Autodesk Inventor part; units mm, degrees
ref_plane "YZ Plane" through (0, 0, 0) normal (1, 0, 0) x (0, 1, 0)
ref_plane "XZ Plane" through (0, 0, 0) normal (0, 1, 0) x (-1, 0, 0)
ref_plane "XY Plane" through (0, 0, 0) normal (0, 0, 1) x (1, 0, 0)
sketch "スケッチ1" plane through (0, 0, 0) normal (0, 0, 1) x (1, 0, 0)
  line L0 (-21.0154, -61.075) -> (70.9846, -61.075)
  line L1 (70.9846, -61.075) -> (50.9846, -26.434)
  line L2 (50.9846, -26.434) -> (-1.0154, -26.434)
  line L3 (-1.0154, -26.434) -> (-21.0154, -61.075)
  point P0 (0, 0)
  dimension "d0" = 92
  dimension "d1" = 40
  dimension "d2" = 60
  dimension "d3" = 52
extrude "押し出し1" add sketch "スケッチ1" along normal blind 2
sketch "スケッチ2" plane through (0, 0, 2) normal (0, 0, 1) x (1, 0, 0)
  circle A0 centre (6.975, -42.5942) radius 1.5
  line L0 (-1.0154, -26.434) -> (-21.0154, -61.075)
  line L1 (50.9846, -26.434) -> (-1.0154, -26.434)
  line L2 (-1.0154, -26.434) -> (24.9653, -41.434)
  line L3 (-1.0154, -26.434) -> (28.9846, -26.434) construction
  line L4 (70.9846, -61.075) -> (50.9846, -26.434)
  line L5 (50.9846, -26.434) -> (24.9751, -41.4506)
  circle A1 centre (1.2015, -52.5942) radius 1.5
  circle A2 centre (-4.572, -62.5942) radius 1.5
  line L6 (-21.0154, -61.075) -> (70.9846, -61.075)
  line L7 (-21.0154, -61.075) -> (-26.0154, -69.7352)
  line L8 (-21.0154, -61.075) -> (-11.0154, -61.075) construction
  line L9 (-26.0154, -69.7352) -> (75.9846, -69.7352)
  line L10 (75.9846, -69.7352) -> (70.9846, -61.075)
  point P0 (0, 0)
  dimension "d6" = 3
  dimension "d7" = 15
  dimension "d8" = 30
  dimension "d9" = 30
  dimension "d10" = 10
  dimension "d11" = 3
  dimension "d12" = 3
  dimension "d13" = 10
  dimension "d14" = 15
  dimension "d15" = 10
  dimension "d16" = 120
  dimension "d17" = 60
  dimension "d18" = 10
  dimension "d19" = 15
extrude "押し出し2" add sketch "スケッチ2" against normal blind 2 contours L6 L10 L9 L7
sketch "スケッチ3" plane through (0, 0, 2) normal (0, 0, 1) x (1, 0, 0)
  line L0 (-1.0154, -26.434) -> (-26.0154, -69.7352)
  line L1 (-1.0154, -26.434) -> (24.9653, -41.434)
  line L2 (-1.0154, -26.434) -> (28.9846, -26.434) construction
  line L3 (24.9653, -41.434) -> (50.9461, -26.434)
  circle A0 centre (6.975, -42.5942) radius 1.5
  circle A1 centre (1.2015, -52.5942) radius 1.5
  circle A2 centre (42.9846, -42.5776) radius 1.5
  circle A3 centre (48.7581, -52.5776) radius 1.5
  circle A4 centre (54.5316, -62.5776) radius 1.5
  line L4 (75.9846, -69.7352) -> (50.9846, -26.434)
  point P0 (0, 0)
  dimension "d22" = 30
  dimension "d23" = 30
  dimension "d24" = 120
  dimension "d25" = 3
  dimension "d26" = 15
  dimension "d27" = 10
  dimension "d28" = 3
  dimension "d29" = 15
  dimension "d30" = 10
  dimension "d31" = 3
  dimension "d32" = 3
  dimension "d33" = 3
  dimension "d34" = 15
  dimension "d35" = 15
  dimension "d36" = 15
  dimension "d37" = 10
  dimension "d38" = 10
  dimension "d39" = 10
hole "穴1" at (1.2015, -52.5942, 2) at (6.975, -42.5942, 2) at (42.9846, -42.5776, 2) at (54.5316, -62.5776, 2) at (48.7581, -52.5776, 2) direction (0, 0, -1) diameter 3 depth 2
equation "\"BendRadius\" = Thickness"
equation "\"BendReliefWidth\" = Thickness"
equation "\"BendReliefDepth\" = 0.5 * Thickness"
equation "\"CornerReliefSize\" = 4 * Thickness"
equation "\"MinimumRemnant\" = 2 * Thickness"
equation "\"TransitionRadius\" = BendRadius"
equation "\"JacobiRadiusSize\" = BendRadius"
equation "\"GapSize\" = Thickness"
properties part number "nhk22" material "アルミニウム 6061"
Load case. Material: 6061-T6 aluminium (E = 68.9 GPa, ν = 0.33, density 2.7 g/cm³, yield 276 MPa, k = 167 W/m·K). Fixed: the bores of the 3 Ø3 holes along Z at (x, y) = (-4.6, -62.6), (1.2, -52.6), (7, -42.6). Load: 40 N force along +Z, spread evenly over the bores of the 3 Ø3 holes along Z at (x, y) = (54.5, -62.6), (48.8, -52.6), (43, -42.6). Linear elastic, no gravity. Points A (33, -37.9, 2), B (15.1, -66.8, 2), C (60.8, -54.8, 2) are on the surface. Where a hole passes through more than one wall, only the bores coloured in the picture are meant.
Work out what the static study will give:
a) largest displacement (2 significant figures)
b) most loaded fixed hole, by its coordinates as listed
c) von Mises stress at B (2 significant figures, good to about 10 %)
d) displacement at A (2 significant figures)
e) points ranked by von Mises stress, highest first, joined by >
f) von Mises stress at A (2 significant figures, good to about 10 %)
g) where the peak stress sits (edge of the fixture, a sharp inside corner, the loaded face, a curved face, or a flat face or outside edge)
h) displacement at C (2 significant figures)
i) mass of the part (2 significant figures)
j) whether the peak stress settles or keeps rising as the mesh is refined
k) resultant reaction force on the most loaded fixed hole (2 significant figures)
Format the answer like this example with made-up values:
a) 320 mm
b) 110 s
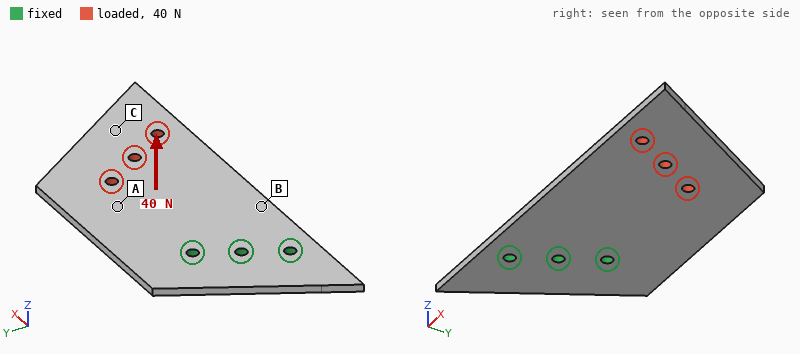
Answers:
a) 1.2 mm
b) (7, -42.6)
c) 40 MPa
d) 0.25 mm
e) B > A > C
f) 22 MPa
g) edge of the fixture
h) 0.83 mm
i) 18 g
j) keeps rising
k) 50 N
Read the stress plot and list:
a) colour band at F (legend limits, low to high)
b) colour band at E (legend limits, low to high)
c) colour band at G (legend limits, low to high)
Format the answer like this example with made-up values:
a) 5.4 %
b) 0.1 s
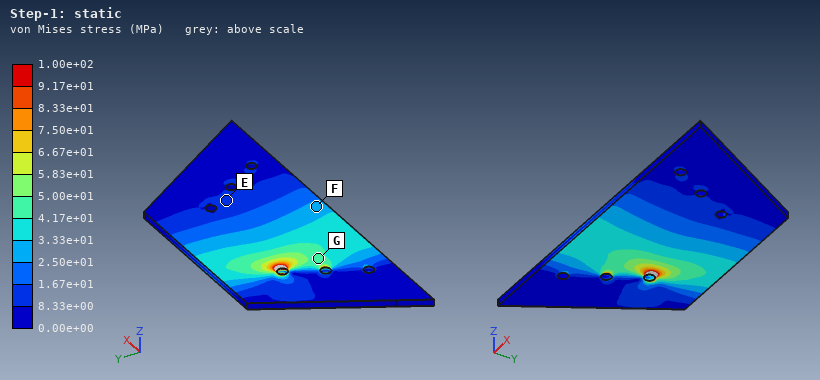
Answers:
a) 2.50e+01 to 3.33e+01 MPa
b) 8.33e+00 to 1.67e+01 MPa
c) 4.17e+01 to 5.00e+01 MPa
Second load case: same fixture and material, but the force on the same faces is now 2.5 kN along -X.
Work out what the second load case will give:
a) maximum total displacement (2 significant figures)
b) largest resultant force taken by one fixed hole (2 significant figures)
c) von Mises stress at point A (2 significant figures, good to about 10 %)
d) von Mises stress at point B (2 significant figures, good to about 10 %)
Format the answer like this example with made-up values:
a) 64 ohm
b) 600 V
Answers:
a) 49 µm
b) 890 N
c) 25 MPa
d) 38 MPa
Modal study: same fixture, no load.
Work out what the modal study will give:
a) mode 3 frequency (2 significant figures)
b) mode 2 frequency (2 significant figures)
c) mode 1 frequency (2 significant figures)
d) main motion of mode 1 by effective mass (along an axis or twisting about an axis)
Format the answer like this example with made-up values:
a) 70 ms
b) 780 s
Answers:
a) 2400 Hz
b) 1400 Hz
c) 450 Hz
d) along Z
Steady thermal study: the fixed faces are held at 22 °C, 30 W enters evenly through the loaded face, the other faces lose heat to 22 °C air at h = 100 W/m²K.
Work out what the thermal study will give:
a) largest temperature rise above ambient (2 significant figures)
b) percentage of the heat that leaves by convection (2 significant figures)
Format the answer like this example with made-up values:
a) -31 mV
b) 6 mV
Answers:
a) 61 K
b) 58 %
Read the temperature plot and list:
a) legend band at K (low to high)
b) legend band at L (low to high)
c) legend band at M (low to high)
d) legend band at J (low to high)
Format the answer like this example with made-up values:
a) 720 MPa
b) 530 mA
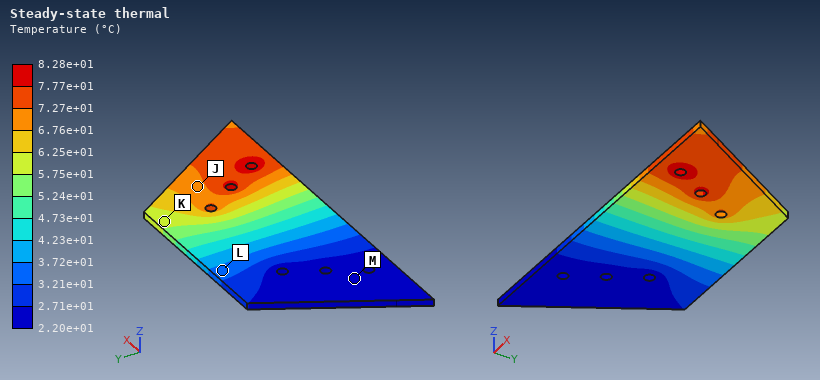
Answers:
a) 5.75e+01 to 6.25e+01 °C
b) 3.21e+01 to 3.72e+01 °C
c) 2.20e+01 to 2.71e+01 °C
d) 6.76e+01 to 7.27e+01 °C
